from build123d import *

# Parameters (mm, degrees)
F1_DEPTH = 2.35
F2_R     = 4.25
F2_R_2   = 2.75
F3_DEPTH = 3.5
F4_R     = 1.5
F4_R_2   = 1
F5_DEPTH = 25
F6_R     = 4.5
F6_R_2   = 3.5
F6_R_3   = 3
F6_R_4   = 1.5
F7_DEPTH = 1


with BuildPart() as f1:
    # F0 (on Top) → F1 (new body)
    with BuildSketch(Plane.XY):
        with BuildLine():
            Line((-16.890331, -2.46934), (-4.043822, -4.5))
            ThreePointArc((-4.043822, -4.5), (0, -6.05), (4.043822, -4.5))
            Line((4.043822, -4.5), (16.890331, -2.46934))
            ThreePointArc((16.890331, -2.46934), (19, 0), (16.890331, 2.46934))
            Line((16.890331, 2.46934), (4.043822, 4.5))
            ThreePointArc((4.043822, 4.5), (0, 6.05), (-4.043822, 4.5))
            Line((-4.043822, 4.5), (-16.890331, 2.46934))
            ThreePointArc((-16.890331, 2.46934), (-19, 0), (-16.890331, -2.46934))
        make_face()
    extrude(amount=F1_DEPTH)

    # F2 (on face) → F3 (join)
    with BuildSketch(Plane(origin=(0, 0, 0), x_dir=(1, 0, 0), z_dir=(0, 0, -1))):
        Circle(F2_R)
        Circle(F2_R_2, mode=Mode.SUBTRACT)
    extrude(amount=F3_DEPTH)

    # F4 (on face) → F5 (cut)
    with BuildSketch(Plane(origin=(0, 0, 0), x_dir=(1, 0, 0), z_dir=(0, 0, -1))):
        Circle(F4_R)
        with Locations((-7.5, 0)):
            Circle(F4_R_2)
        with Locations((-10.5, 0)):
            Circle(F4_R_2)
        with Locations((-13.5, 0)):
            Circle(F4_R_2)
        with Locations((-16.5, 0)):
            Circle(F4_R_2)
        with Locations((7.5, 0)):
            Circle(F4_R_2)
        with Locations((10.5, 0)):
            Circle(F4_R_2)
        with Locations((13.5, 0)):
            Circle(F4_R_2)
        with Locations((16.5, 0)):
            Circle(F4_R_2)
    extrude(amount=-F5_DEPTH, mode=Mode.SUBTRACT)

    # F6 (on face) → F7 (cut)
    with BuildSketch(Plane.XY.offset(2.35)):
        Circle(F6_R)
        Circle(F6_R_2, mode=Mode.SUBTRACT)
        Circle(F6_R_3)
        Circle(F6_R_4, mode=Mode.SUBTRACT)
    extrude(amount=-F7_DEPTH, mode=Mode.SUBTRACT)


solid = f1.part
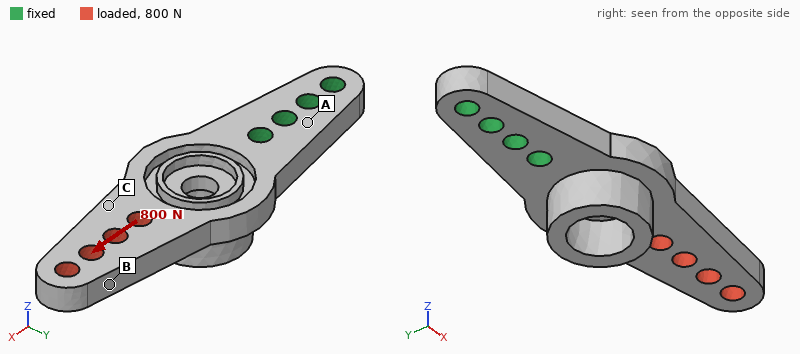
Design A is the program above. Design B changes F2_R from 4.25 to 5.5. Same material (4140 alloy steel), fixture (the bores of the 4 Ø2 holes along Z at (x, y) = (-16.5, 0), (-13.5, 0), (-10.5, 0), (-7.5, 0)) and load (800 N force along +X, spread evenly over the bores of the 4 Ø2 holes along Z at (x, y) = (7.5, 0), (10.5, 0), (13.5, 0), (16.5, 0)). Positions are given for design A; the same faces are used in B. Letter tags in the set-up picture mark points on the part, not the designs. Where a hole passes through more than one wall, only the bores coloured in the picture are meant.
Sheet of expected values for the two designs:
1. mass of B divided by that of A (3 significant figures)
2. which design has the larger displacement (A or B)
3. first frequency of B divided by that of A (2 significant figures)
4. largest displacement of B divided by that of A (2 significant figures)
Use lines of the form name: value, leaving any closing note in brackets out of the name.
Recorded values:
mass of B divided by that of A: 1.20
which design has the larger displacement: A
first frequency of B divided by that of A: 1.2
largest displacement of B divided by that of A: 0.73
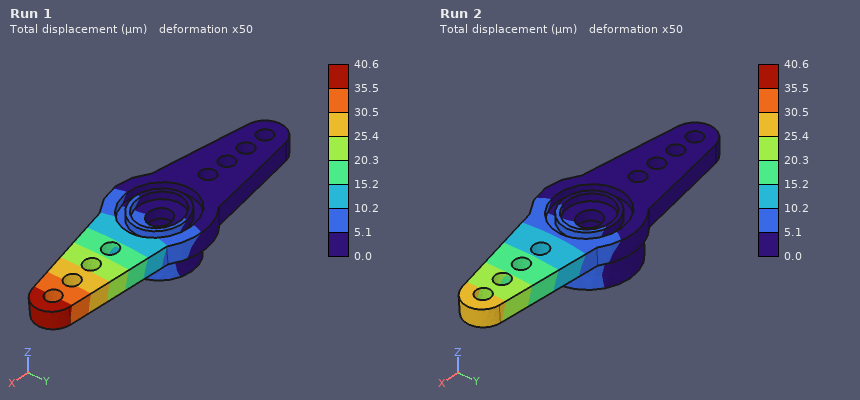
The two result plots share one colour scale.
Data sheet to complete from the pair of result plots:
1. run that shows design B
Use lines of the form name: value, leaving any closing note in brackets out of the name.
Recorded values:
run that shows design B: Run 2
